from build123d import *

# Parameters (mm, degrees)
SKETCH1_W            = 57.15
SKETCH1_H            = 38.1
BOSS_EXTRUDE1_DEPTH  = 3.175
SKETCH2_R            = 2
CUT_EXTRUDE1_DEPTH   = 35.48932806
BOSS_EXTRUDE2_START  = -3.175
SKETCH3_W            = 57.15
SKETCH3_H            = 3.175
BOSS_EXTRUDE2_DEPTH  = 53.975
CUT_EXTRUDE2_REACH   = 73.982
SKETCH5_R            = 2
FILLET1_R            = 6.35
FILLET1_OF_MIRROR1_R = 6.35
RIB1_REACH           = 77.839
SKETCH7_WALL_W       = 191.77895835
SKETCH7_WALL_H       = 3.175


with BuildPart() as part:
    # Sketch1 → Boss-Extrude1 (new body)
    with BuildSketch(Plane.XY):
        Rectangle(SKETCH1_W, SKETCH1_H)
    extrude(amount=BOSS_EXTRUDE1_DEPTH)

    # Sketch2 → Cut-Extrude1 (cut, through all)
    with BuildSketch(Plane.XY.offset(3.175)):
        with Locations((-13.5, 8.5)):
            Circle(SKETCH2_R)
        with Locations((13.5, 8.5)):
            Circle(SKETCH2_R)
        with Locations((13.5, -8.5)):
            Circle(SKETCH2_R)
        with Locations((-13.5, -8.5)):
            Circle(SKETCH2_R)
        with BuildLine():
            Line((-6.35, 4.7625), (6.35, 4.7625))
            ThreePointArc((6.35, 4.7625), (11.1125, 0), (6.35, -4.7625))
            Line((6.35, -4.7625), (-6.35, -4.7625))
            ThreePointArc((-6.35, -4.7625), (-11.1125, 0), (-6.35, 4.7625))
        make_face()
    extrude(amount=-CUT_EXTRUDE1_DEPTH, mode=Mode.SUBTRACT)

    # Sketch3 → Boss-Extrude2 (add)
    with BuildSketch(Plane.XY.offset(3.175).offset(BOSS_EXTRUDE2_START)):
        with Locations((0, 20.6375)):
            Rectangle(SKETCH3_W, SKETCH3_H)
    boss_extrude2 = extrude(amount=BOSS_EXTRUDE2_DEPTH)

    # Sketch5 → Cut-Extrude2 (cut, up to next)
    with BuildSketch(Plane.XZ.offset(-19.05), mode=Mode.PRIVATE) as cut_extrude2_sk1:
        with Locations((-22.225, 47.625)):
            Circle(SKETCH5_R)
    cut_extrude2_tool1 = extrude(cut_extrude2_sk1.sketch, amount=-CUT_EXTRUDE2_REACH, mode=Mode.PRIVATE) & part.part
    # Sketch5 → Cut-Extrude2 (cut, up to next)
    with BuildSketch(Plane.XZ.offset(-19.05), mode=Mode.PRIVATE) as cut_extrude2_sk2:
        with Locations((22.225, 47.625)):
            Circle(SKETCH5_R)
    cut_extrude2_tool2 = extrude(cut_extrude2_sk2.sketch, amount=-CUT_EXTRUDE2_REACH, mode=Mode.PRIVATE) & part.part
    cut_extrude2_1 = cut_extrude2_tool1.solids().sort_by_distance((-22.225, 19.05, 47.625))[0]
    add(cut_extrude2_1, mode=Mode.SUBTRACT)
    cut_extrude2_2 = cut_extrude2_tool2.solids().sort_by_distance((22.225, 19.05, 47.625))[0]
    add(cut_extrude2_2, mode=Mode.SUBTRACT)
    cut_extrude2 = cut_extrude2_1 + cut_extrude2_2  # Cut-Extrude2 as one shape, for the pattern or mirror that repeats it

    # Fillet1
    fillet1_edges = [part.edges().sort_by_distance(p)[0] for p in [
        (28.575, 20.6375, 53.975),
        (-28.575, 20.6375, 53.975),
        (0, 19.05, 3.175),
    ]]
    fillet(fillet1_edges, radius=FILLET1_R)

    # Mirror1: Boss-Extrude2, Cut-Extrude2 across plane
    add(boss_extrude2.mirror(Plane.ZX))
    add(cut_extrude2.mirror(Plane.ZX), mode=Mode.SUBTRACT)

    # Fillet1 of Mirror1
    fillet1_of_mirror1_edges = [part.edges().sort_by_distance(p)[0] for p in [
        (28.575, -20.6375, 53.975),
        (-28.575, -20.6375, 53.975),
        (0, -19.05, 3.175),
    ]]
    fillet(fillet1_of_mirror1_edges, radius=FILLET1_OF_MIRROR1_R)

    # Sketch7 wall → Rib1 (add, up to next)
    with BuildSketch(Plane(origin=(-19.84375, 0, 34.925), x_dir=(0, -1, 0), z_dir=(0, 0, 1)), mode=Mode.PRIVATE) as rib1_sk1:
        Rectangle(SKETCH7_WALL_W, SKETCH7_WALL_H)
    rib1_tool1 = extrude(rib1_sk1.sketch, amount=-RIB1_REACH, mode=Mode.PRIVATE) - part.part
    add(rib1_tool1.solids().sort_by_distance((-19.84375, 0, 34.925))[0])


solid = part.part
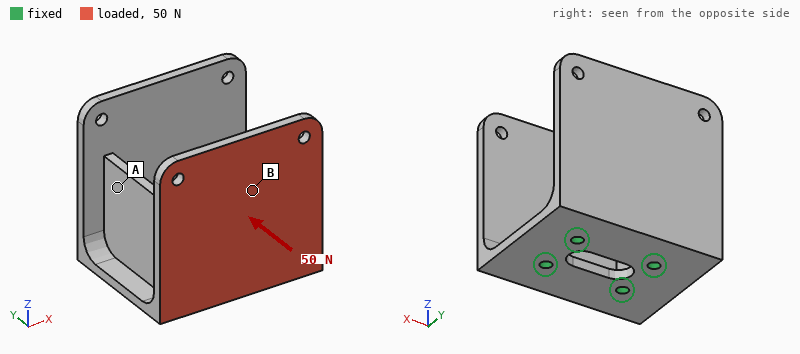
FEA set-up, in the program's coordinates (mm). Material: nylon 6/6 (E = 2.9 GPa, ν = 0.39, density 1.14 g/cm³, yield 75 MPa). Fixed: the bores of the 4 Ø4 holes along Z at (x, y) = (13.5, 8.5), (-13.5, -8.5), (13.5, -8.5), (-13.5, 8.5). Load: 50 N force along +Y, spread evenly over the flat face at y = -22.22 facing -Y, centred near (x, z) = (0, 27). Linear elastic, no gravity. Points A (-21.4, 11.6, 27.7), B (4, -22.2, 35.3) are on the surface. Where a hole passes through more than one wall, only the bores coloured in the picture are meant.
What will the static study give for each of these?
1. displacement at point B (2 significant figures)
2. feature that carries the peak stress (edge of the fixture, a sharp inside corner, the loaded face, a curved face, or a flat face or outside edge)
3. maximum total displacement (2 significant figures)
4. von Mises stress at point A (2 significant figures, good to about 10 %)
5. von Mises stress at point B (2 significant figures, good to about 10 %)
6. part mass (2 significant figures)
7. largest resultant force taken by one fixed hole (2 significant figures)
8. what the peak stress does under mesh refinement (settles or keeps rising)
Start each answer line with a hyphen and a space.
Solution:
- 0.39 mm
- edge of the fixture
- 0.98 mm
- 0.81 MPa
- 2.2 MPa
- 34 g
- 54 N
- keeps rising
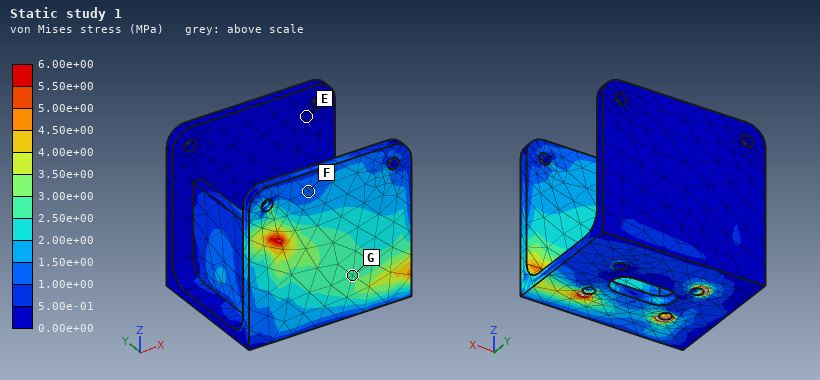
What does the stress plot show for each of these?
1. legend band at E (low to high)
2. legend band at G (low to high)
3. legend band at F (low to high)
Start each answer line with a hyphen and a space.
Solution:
- 0.00e+00 to 5.00e-01 MPa
- 2.50e+00 to 3.00e+00 MPa
- 1.00e+00 to 1.50e+00 MPa
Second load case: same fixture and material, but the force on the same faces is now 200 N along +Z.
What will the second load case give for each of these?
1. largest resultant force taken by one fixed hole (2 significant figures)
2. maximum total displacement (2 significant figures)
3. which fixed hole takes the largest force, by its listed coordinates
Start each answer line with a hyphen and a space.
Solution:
- 180 N
- 0.97 mm
- (-13.5, -8.5)
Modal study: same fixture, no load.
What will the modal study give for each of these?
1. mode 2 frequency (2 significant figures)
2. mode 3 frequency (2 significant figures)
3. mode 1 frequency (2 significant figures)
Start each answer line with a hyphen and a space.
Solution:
- 470 Hz
- 830 Hz
- 470 Hz
